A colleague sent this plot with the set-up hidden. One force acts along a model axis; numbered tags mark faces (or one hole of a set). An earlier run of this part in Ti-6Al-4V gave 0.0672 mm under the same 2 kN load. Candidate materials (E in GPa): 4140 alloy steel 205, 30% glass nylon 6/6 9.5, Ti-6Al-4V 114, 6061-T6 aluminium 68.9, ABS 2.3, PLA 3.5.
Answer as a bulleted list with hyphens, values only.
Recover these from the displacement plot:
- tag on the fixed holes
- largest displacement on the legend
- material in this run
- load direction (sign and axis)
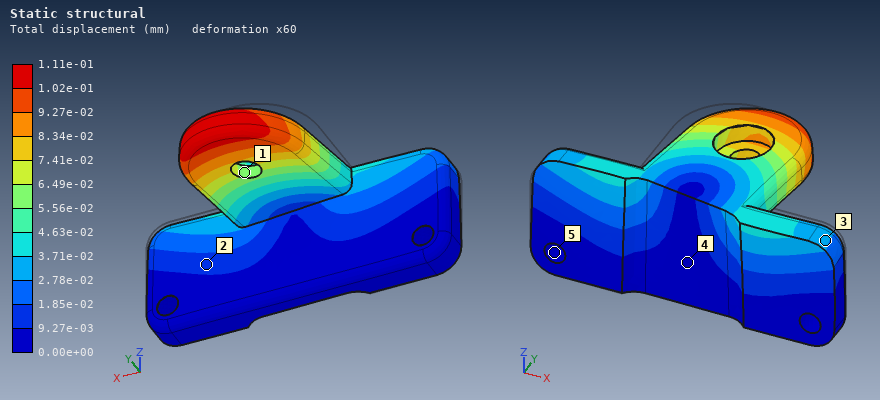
- 5
- 1.11e-01 mm
- 6061-T6 aluminium
- +X
